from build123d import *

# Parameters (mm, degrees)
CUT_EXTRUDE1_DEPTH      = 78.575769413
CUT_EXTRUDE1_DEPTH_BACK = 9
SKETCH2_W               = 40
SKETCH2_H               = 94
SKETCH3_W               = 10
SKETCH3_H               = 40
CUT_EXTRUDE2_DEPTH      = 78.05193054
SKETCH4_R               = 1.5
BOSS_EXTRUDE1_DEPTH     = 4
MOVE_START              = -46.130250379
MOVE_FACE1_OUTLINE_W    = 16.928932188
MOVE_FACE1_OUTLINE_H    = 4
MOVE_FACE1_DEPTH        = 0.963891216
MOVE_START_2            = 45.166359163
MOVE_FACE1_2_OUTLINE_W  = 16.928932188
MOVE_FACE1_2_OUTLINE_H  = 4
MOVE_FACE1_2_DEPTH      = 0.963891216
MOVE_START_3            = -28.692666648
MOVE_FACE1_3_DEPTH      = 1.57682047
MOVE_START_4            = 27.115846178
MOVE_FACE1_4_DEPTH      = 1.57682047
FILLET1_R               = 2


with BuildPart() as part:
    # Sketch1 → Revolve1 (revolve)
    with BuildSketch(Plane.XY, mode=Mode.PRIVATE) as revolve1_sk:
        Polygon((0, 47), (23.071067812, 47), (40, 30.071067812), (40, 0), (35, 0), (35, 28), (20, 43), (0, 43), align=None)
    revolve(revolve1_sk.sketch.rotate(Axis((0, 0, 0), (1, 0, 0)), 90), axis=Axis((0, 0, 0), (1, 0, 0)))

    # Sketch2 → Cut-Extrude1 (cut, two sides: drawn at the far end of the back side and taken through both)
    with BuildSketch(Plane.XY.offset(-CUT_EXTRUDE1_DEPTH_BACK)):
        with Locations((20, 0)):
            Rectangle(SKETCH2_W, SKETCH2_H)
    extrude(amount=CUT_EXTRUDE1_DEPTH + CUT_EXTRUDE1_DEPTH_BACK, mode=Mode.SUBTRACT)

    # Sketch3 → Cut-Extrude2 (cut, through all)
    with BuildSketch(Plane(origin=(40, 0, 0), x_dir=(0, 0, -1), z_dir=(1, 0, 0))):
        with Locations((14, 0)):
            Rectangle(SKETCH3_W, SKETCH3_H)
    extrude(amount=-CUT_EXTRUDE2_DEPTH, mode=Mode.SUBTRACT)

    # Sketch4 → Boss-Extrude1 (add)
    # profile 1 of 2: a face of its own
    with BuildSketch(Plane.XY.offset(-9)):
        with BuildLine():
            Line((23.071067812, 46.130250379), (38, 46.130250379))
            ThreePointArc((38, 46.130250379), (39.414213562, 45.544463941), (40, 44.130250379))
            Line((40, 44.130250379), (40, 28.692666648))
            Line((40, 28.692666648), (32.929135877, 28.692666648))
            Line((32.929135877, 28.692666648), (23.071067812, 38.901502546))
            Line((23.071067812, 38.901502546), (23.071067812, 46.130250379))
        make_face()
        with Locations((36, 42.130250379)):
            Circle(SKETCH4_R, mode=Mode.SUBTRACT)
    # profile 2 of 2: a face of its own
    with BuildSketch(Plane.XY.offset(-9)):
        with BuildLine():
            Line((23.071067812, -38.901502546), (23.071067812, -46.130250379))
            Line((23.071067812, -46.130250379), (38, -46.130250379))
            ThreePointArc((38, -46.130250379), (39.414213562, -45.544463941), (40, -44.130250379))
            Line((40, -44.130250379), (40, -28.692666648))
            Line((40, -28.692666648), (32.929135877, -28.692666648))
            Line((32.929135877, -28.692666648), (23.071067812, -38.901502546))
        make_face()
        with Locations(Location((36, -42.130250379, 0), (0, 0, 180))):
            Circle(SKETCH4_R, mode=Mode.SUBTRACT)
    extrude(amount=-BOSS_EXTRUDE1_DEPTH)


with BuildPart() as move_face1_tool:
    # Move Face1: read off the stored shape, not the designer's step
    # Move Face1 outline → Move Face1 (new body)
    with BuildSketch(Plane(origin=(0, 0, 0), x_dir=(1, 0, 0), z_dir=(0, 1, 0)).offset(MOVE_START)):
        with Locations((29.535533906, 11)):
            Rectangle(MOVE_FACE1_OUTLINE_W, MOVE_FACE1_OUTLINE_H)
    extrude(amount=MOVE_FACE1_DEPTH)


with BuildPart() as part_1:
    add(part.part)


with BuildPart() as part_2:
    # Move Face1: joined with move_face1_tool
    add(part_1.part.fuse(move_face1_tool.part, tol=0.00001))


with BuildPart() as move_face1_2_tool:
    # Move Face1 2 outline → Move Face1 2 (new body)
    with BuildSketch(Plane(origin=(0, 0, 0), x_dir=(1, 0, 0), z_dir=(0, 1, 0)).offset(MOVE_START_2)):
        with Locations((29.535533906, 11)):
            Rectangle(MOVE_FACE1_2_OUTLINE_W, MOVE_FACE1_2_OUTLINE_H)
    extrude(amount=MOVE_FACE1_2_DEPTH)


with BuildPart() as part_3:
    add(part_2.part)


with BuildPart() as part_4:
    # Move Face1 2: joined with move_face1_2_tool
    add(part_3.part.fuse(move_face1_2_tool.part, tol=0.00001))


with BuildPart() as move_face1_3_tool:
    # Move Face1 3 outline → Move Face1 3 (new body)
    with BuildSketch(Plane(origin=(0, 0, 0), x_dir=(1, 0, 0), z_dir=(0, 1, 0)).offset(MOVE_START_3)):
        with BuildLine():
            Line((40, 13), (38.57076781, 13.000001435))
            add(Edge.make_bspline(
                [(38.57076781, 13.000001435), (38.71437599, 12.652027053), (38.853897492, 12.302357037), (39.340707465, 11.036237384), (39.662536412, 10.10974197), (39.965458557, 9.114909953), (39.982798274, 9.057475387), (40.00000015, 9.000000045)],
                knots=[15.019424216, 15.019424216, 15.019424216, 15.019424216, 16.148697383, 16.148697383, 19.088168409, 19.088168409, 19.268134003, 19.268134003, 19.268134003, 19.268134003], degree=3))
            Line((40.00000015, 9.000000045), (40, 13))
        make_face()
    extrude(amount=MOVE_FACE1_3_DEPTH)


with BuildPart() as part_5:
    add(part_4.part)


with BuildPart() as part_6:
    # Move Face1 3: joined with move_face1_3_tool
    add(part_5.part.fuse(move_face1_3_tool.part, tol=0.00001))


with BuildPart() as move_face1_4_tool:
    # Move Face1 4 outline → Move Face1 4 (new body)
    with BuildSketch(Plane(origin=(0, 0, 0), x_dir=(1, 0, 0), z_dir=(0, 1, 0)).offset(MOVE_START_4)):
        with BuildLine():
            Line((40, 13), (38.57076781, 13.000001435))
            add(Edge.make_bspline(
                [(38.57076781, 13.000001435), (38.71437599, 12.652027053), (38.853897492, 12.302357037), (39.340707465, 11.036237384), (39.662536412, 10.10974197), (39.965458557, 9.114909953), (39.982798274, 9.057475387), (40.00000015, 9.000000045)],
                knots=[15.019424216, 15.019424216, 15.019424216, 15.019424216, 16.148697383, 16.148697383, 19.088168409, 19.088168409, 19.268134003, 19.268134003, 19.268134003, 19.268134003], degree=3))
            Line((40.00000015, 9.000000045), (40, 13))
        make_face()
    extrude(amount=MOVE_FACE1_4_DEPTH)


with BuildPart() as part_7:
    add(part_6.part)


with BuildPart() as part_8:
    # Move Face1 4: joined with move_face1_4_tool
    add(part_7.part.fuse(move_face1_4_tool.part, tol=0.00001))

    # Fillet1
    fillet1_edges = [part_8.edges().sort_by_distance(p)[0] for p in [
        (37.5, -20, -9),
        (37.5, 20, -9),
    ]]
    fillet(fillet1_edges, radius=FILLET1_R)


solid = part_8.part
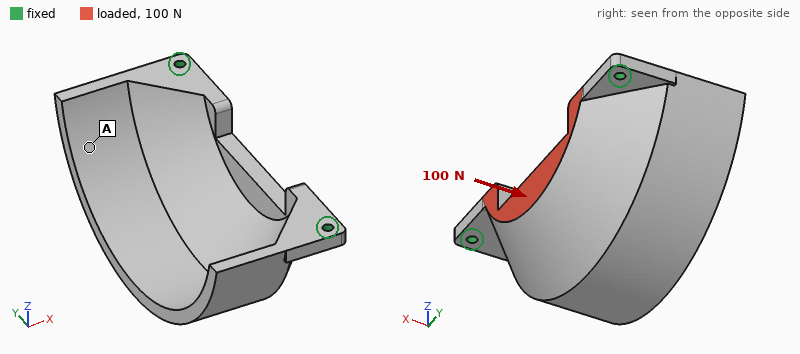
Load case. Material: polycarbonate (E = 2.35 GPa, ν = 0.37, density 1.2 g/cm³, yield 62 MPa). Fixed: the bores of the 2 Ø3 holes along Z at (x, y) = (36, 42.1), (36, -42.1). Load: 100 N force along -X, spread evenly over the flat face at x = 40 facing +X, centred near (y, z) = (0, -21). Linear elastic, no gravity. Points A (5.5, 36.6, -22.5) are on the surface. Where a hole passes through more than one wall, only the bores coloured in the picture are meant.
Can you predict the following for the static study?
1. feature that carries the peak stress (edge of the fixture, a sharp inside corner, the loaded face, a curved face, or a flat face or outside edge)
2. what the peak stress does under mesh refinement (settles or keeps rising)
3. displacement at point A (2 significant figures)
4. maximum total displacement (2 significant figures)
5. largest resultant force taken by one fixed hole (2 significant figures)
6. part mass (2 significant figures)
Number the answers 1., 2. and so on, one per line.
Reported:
1. edge of the fixture
2. keeps rising
3. 0.66 mm
4. 1.2 mm
5. 57 N
6. 30 g
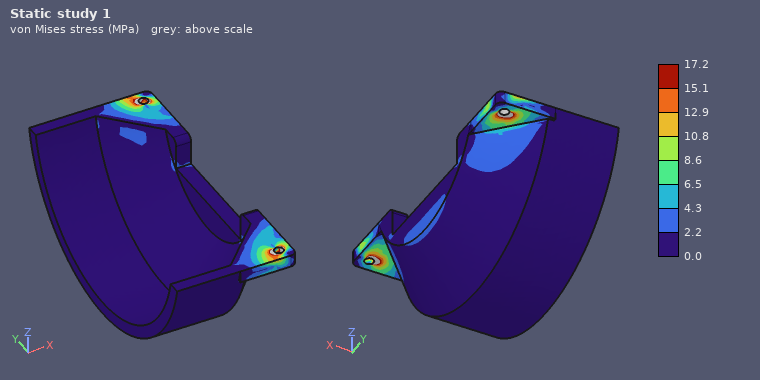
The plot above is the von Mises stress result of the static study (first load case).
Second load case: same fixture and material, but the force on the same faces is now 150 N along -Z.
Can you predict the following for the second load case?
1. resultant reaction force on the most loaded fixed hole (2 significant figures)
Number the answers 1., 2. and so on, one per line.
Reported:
1. 120 N
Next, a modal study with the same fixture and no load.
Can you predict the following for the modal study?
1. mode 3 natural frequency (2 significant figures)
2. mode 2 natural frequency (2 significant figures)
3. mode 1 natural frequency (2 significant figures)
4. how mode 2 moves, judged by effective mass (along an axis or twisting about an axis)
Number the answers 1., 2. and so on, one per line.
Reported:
1. 1200 Hz
2. 670 Hz
3. 240 Hz
4. along Y
